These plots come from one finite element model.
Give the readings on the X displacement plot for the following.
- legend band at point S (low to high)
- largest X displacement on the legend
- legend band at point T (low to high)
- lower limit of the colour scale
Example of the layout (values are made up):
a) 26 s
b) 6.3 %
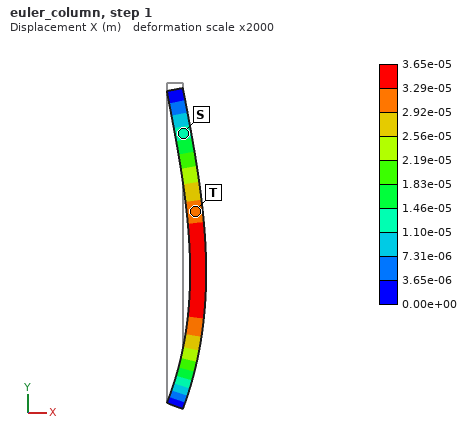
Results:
a) 1.10e-05 to 1.46e-05 m
b) 3.65e-05 m
c) 2.92e-05 to 3.29e-05 m
d) 0.00e+00 m
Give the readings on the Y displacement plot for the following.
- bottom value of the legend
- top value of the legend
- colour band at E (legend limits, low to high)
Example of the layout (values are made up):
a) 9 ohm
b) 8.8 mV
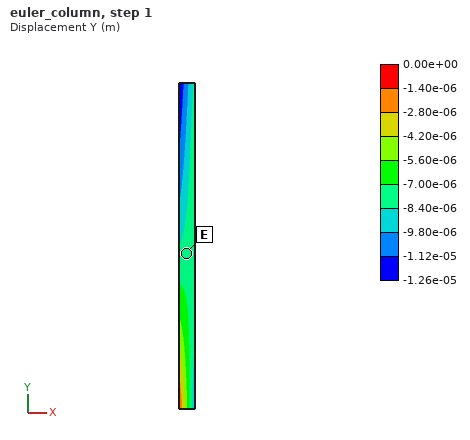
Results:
a) -1.26e-05 m
b) 0.00e+00 m
c) -8.40e-06 to -7.00e-06 m
